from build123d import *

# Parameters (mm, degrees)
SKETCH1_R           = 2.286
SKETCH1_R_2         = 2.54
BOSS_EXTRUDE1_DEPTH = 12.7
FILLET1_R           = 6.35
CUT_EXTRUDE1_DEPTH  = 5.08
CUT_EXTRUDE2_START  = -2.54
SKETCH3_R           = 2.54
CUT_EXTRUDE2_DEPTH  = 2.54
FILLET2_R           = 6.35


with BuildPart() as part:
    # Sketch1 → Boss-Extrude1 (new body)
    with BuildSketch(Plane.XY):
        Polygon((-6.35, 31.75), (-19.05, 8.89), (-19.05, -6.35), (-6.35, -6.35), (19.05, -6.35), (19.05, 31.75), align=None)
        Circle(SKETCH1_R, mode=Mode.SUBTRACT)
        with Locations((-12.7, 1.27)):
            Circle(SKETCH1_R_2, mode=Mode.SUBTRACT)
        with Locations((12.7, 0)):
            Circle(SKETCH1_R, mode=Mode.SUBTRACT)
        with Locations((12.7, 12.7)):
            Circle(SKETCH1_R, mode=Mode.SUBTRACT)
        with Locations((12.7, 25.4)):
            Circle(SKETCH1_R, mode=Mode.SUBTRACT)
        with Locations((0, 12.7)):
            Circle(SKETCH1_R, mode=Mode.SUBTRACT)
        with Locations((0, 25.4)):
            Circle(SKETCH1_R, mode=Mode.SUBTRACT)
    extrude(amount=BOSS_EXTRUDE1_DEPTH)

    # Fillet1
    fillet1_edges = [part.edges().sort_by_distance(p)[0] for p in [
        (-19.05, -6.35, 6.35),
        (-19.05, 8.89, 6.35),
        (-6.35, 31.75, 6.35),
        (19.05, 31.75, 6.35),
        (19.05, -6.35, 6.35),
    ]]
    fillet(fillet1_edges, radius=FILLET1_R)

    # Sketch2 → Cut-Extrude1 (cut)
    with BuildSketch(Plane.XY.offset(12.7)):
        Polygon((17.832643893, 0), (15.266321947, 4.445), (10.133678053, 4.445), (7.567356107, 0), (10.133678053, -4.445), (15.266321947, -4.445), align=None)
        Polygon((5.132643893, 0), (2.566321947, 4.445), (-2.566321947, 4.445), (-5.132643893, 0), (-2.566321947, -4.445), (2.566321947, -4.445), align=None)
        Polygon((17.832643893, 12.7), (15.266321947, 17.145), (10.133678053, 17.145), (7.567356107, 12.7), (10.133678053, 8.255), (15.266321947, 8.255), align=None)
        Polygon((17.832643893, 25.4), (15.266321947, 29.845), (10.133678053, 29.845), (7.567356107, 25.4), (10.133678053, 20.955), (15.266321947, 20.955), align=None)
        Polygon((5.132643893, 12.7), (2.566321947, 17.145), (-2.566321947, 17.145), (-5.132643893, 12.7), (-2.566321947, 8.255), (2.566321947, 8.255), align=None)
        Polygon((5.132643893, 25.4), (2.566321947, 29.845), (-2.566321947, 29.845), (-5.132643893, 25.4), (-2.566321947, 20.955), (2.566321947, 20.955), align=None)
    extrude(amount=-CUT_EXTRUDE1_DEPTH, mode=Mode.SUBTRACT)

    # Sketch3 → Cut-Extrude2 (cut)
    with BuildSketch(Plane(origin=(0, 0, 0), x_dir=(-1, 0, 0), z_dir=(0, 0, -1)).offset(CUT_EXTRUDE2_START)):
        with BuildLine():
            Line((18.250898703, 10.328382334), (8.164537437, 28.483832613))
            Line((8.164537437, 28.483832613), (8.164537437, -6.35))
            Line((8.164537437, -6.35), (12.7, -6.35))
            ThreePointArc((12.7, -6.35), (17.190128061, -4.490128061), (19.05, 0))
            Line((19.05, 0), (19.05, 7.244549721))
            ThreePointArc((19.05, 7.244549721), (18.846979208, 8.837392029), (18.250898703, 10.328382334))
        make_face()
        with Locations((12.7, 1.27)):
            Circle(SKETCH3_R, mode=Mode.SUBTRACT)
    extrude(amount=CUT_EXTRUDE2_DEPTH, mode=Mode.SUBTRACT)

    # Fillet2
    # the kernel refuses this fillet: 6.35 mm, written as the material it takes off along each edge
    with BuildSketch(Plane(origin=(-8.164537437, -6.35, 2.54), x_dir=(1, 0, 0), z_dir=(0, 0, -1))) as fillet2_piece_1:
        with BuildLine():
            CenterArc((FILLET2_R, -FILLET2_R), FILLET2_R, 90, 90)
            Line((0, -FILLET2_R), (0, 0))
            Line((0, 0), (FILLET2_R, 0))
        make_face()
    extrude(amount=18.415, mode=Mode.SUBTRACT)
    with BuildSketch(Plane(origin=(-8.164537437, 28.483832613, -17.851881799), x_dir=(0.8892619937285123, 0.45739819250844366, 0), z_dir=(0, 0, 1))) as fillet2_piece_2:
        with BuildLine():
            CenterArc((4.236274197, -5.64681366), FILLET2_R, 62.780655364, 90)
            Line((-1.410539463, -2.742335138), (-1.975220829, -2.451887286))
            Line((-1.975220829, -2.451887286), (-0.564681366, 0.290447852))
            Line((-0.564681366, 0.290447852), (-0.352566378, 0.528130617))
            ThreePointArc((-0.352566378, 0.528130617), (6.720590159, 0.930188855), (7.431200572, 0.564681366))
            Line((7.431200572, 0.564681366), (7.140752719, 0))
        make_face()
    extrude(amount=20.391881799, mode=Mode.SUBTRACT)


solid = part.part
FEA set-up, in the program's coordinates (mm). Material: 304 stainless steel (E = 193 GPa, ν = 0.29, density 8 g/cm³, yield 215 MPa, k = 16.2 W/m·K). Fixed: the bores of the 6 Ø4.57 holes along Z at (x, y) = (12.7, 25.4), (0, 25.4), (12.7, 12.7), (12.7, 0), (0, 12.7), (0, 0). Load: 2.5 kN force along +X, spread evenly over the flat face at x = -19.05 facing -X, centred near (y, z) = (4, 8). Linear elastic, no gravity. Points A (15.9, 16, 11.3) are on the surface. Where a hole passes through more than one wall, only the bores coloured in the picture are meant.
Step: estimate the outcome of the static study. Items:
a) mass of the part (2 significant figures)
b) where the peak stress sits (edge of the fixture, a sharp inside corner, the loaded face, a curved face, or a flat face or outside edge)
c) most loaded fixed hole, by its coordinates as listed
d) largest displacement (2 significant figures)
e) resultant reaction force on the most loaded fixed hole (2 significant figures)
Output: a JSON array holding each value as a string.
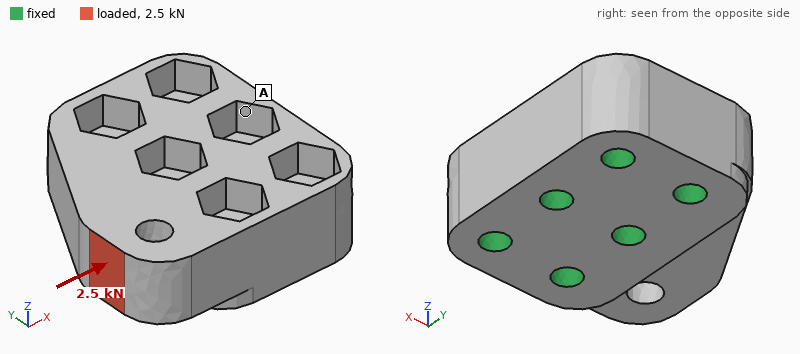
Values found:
["100 g", "a curved face", "(0, 0)", "5.0 µm", "1.3 kN"]
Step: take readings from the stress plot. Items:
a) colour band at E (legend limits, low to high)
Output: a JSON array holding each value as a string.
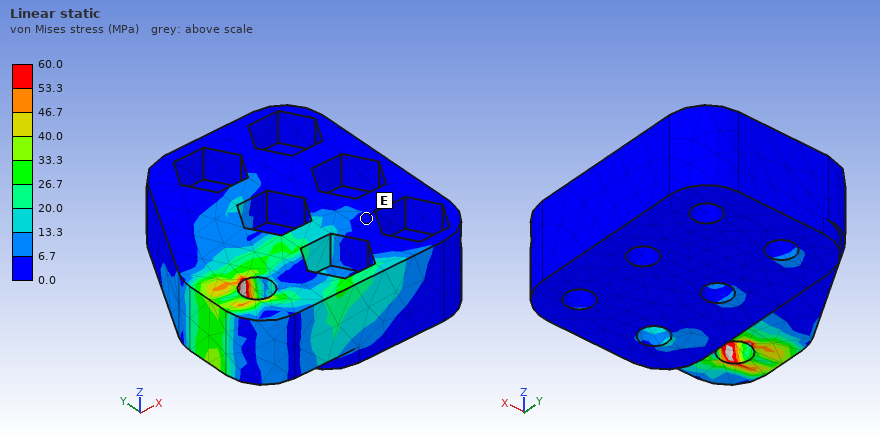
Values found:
["0.0 to 6.7 MPa"]
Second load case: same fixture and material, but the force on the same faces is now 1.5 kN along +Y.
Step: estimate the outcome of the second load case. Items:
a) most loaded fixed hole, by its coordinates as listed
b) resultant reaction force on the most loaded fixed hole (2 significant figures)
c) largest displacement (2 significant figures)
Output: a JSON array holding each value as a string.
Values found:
["(0, 0)", "1.1 kN", "3.4 µm"]
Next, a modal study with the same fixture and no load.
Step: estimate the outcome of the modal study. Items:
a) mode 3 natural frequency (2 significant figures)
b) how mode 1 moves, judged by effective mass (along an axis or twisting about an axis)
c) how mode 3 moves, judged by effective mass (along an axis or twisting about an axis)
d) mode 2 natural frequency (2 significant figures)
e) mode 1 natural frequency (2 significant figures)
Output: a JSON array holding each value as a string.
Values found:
["37 kHz", "along Z", "along Y", "35 kHz", "20 kHz"]
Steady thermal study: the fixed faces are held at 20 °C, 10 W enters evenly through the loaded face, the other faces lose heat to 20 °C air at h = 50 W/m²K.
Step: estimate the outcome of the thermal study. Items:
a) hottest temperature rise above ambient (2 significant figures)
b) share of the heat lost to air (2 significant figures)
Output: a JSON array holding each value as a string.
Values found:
["71 K", "19 %"]
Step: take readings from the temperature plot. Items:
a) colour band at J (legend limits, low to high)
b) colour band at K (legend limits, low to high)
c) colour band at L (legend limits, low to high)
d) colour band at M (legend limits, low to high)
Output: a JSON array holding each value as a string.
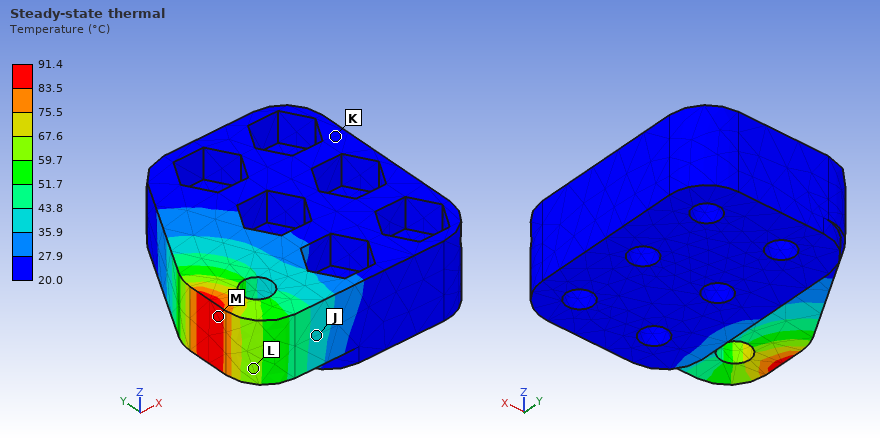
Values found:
["35.9 to 43.8 °C", "20.0 to 27.9 °C", "59.7 to 67.6 °C", "83.5 to 91.4 °C"]
